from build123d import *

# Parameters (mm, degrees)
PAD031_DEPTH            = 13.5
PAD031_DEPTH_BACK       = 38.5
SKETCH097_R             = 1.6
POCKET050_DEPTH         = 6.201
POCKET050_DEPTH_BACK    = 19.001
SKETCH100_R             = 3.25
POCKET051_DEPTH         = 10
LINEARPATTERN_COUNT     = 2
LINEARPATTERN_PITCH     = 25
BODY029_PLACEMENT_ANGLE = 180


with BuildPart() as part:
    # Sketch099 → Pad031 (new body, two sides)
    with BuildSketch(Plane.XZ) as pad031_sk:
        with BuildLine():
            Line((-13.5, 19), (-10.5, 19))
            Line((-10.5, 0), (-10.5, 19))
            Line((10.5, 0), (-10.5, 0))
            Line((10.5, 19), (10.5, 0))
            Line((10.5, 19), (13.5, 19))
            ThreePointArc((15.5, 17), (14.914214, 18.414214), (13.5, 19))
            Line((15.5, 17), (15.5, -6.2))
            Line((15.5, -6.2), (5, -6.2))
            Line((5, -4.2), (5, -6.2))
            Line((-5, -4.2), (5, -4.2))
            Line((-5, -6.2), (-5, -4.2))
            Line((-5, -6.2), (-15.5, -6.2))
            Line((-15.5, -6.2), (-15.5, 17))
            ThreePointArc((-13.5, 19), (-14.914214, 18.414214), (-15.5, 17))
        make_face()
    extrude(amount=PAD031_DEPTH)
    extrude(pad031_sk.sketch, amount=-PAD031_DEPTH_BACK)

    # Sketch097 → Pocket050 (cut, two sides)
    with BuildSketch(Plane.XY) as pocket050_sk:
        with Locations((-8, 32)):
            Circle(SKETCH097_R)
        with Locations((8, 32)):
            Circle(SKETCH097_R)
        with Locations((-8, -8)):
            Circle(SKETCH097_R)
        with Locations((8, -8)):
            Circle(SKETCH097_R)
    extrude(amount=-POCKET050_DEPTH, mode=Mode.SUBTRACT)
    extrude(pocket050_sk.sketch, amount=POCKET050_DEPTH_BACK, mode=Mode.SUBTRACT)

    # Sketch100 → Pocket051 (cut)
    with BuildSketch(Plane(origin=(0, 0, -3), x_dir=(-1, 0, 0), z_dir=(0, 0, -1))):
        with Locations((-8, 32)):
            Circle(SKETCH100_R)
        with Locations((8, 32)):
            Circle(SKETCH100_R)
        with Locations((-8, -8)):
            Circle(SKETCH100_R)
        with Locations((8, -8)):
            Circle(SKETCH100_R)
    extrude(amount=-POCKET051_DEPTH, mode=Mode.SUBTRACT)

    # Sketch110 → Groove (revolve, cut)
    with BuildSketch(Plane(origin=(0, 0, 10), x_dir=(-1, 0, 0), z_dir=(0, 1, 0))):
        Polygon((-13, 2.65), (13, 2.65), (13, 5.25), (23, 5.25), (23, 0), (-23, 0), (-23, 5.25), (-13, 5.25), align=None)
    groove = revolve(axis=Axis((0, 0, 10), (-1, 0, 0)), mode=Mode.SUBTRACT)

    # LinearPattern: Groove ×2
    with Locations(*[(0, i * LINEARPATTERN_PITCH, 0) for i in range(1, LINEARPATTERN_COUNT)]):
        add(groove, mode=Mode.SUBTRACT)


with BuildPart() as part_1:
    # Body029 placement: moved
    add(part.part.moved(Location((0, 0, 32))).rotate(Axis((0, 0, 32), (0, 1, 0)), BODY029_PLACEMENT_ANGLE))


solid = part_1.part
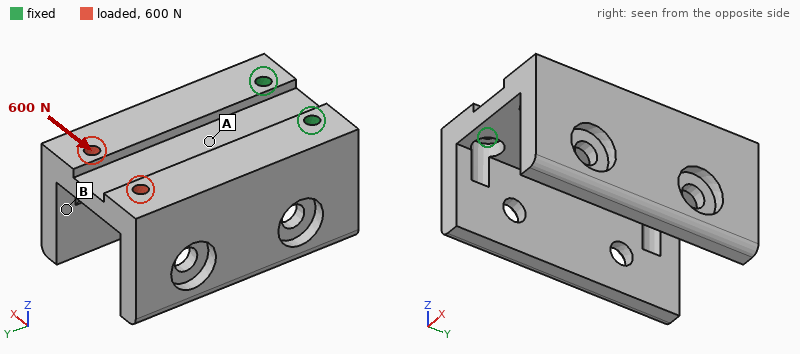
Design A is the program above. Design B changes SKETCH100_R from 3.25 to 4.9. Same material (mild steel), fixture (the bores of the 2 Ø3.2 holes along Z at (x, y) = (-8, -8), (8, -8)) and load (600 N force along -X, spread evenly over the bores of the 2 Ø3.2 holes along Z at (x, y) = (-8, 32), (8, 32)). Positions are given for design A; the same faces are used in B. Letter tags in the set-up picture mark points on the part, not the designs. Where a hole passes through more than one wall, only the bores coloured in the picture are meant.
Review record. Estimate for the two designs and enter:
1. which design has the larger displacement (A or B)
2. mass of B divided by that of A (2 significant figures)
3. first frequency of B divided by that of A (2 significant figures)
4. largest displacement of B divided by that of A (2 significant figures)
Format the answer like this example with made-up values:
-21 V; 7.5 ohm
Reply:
B; 0.95; 0.93; 1.1
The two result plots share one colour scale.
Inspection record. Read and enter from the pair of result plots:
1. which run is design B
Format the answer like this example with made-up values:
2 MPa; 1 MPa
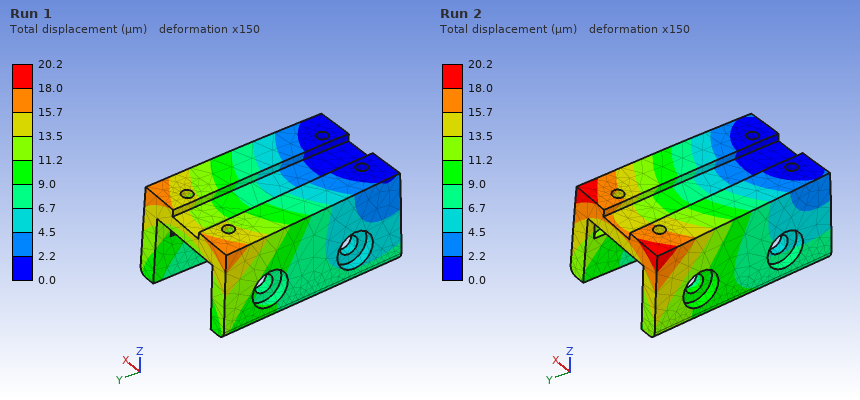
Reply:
Run 2
